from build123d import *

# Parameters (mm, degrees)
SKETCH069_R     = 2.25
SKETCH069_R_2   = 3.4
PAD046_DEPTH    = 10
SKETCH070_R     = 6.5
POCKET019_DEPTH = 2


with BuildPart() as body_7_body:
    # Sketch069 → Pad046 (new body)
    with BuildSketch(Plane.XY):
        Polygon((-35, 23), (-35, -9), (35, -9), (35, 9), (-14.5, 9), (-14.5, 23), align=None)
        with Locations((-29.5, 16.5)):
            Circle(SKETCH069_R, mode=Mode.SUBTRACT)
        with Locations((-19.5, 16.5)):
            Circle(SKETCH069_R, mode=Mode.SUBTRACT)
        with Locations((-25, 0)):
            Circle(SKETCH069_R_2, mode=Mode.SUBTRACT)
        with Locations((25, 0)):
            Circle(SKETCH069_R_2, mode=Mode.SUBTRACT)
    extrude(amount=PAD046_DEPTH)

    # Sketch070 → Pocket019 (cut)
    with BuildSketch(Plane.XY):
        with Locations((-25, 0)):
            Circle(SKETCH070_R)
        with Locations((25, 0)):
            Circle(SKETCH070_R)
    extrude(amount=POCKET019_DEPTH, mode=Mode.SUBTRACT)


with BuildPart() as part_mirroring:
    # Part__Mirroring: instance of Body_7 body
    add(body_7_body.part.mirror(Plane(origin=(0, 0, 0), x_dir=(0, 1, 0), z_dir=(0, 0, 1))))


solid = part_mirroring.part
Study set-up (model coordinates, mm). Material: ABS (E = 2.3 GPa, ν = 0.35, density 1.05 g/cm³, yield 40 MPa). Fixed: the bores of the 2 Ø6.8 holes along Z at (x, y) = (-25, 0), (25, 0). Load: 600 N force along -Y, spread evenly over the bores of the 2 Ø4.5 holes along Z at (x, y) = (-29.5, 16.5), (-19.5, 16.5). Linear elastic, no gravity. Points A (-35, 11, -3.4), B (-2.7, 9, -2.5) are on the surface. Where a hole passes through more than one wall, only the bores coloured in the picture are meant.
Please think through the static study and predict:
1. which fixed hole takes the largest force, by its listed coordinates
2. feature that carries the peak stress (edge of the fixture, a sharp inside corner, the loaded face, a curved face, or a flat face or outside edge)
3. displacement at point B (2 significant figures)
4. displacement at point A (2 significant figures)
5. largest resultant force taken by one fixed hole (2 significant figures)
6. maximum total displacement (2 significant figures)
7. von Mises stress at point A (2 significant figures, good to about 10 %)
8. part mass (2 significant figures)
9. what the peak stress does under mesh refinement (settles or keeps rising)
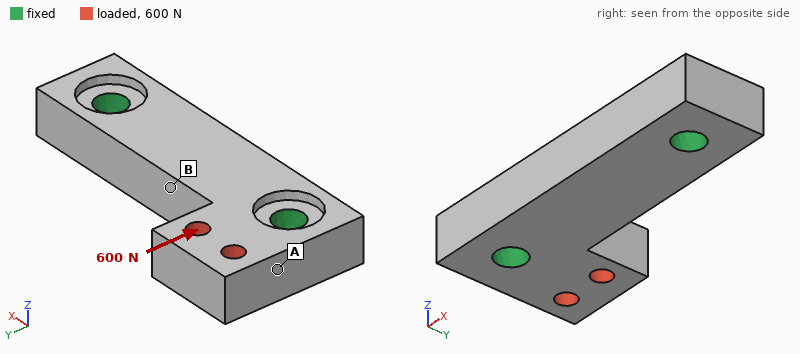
(-25, 0)
edge of the fixture
10 µm
26 µm
590 N
44 µm
2.3 MPa
15 g
keeps rising
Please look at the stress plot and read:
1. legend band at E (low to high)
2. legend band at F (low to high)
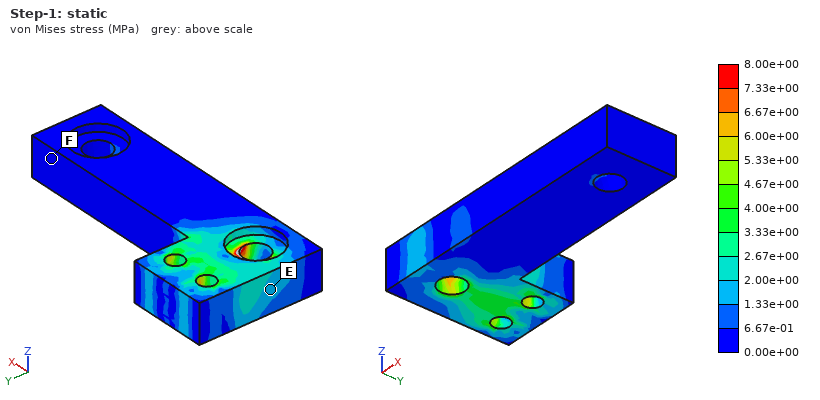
1.33e+00 to 2.00e+00 MPa
0.00e+00 to 6.67e-01 MPa
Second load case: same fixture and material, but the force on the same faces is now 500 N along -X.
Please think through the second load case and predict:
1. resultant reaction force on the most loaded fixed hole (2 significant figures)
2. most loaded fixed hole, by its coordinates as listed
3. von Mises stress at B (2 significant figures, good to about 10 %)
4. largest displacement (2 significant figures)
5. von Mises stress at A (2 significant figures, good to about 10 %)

420 N
(-25, 0)
3.5 MPa
0.19 mm
4.5 MPa
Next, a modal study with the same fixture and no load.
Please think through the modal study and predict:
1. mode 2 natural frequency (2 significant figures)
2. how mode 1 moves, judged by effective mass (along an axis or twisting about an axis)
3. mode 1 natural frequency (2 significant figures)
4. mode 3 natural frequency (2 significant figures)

4800 Hz
along Z
3900 Hz
4900 Hz
